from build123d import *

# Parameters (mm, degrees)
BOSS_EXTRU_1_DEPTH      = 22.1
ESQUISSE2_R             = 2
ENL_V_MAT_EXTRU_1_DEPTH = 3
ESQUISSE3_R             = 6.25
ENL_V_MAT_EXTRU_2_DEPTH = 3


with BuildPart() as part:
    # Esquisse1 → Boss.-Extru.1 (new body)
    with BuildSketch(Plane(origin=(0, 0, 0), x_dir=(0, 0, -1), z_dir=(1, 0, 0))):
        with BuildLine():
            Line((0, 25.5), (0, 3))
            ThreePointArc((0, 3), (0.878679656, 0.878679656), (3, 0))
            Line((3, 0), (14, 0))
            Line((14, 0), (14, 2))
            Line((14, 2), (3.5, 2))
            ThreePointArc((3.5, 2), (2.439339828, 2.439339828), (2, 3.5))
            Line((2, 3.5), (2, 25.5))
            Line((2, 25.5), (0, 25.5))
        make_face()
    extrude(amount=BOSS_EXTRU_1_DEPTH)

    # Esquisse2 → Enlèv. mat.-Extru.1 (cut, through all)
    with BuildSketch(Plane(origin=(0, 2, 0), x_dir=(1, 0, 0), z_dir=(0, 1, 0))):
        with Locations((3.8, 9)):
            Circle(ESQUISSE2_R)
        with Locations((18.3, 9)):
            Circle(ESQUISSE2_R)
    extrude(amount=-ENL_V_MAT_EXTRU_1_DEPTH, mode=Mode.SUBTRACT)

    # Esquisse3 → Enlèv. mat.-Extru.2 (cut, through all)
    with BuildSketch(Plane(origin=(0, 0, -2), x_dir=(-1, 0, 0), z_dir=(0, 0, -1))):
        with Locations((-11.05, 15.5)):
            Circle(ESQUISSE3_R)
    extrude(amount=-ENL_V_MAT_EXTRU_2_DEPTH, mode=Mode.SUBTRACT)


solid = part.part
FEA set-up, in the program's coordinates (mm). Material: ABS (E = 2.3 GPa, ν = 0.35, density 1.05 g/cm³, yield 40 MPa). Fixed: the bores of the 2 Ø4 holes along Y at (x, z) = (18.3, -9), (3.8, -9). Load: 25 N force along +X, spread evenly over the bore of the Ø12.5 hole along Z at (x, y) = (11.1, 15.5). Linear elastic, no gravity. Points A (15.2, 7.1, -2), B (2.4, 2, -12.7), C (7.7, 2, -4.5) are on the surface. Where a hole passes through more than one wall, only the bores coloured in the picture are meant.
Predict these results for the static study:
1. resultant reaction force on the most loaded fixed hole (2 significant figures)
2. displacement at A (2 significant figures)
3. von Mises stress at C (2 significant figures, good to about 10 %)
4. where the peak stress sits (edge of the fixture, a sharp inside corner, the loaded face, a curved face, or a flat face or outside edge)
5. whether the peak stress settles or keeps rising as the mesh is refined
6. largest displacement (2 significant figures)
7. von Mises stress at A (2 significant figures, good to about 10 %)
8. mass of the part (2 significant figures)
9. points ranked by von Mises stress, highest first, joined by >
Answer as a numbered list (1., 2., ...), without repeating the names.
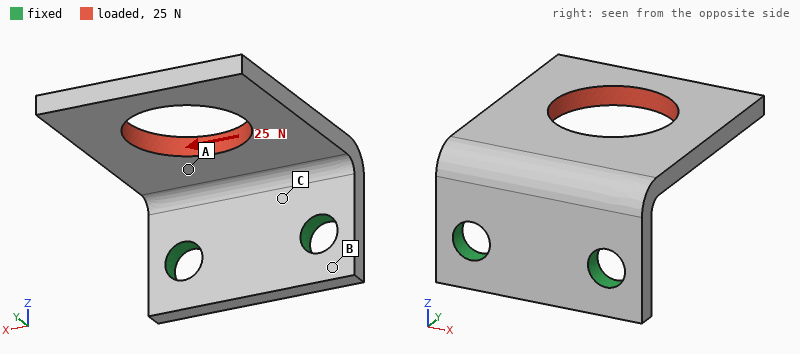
1. 28 N
2. 0.096 mm
3. 6.7 MPa
4. edge of the fixture
5. keeps rising
6. 0.39 mm
7. 3.6 MPa
8. 1.4 g
9. C > A > B
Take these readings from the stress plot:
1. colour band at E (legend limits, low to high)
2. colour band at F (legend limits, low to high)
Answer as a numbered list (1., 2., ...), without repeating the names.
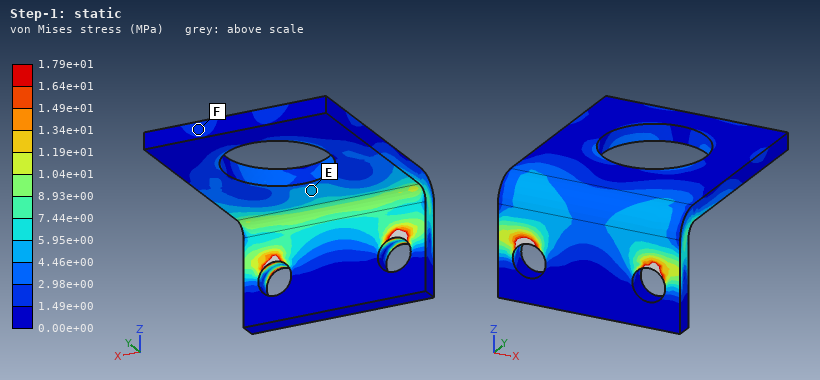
1. 4.46e+00 to 5.95e+00 MPa
2. 1.49e+00 to 2.98e+00 MPa
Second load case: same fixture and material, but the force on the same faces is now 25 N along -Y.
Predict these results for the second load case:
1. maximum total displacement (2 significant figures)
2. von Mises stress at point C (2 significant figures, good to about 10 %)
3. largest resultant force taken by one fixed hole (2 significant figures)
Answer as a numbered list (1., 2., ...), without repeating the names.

1. 0.42 mm
2. 4.7 MPa
3. 13 N
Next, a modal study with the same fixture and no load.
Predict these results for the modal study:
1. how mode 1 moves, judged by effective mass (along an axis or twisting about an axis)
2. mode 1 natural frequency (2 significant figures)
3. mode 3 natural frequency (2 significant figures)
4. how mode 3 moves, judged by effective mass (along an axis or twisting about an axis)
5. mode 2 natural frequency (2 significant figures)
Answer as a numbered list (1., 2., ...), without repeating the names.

1. along Z
2. 630 Hz
3. 2100 Hz
4. along X
5. 1500 Hz
